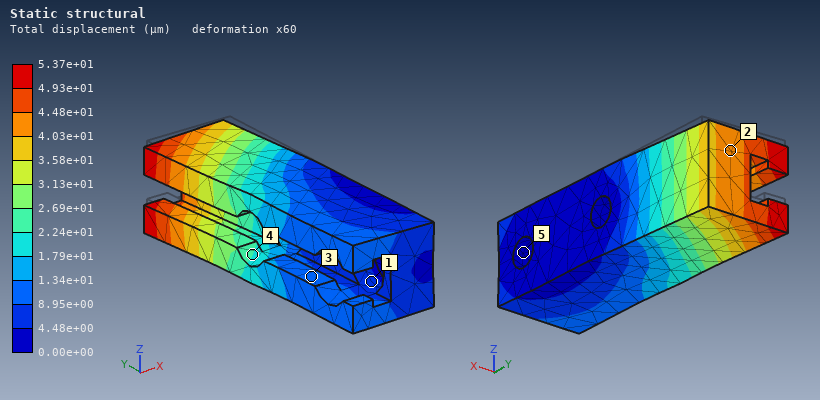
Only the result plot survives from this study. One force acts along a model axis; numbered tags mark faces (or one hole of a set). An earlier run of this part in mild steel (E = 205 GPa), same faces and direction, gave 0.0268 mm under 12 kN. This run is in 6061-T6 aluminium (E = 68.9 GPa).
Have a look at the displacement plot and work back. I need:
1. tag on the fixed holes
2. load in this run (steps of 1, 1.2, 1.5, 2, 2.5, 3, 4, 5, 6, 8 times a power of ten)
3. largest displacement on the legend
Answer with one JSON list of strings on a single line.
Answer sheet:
["5", "8 kN", "5.37e+01 µm"]
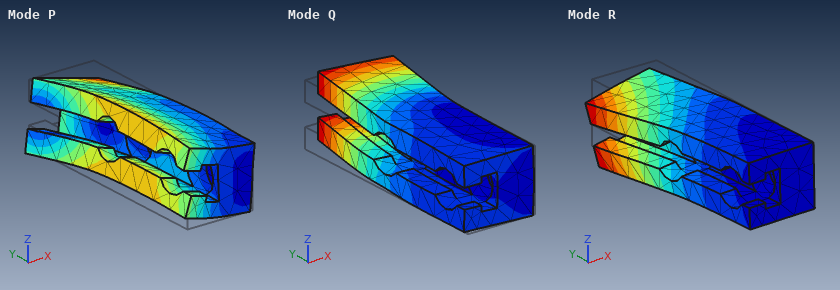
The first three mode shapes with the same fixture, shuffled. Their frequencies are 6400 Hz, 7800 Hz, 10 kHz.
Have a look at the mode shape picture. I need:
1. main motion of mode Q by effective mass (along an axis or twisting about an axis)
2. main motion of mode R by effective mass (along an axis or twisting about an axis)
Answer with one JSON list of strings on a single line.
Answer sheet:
["along X", "along Z"]
